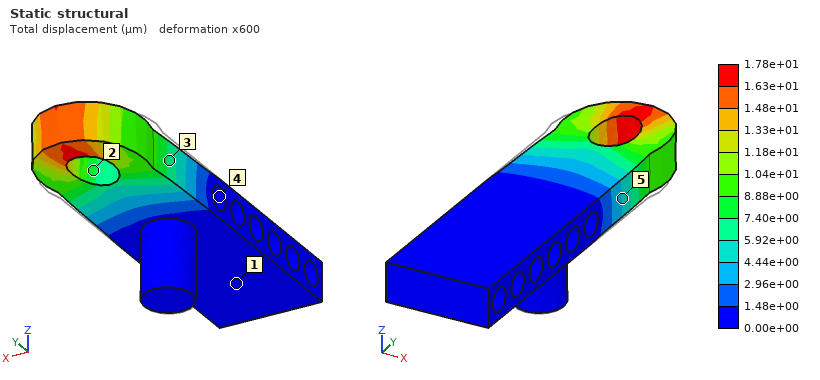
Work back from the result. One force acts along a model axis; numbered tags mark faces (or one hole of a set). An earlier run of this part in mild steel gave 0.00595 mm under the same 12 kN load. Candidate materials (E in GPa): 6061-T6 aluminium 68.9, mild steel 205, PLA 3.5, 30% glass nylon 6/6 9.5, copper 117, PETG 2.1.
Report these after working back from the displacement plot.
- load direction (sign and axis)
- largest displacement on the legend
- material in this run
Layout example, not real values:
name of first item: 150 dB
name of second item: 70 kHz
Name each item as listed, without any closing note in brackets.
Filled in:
load direction: +Y
largest displacement on the legend: 1.78e+01 µm
material in this run: 6061-T6 aluminium
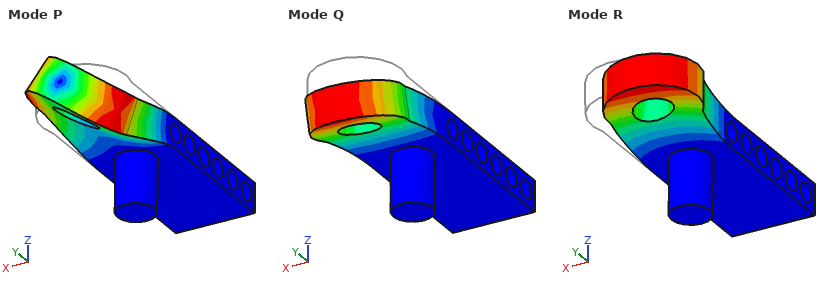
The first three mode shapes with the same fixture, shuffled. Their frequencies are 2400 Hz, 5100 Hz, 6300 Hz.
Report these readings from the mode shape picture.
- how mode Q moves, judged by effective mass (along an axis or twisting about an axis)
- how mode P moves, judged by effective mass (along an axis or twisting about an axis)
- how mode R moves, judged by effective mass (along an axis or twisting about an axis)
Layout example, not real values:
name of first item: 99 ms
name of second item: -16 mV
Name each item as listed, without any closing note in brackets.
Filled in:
how mode Q moves, judged by effective mass: along Z
how mode P moves, judged by effective mass: twisting about Y
how mode R moves, judged by effective mass: along X
